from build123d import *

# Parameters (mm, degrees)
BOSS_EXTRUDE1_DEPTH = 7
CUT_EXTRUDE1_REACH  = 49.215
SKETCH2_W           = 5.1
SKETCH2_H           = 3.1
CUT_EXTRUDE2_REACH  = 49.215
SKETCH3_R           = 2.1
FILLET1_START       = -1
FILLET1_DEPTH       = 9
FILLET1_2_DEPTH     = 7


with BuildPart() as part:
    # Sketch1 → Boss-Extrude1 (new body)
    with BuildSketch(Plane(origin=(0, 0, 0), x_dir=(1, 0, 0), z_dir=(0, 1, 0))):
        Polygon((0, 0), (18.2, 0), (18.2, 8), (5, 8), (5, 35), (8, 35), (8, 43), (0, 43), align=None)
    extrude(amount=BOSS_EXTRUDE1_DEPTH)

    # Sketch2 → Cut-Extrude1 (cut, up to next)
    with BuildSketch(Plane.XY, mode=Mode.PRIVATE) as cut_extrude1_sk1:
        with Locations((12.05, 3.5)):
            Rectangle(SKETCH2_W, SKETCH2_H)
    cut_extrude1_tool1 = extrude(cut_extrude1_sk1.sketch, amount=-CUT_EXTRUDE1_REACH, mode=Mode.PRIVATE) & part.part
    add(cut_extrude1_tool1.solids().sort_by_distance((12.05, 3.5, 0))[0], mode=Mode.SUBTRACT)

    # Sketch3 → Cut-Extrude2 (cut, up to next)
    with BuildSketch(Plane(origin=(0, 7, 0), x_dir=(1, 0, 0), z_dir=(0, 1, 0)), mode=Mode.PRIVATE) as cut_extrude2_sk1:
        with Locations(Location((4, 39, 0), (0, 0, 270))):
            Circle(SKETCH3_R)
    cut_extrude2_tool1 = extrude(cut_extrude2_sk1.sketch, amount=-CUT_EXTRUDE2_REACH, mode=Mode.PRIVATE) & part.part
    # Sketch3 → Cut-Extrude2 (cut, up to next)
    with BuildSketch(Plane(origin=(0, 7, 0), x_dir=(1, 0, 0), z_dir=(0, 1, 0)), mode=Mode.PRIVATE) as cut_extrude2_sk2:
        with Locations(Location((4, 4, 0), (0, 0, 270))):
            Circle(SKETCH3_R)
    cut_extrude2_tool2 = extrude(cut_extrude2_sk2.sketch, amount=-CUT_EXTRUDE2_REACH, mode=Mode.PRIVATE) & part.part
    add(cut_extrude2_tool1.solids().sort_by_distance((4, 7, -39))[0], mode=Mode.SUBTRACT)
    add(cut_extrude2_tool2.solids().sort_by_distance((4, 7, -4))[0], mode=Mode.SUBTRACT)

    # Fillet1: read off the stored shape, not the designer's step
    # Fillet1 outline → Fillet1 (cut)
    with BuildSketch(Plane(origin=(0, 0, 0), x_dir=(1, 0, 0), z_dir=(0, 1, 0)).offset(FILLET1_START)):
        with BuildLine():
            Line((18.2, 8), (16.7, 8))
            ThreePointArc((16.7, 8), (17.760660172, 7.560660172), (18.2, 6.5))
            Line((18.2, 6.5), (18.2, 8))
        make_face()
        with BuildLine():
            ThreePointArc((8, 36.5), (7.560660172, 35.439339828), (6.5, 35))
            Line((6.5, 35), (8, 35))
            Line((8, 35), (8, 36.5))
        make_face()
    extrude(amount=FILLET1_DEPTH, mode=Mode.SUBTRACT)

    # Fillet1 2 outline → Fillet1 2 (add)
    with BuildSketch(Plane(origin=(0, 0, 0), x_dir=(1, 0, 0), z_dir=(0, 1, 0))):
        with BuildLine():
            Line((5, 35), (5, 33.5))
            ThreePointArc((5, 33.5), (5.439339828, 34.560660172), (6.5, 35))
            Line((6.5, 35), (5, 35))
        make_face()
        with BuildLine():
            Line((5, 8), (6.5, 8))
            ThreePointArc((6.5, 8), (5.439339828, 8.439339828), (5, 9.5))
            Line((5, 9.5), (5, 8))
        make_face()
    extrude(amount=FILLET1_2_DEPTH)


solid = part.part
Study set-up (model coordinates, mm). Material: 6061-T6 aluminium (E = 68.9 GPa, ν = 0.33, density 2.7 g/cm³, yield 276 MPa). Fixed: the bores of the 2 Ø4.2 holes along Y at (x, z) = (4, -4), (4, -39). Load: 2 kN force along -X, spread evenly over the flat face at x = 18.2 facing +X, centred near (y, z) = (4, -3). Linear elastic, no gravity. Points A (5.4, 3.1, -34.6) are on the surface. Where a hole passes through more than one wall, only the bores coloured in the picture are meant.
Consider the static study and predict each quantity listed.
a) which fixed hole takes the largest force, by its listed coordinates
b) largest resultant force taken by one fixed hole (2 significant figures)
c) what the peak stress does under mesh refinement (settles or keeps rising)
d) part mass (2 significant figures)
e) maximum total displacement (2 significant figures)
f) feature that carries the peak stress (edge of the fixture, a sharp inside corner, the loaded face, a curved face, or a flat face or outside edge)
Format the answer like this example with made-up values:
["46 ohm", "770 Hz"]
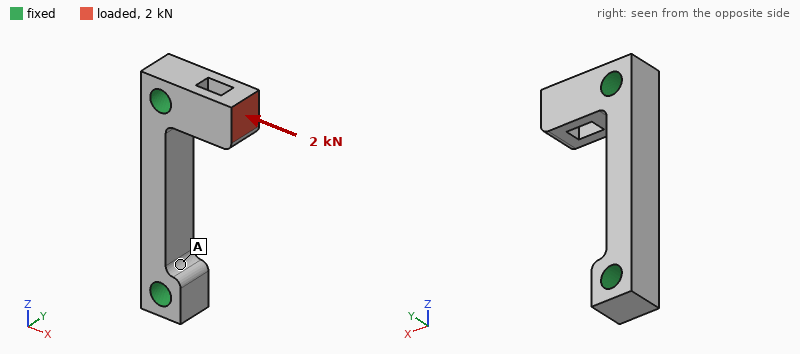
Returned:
["(4, -4)", "2.0 kN", "keeps rising", "5.6 g", "21 µm", "a sharp inside corner"]
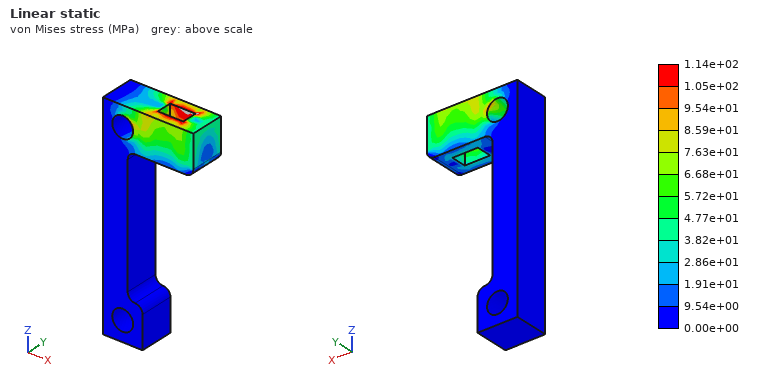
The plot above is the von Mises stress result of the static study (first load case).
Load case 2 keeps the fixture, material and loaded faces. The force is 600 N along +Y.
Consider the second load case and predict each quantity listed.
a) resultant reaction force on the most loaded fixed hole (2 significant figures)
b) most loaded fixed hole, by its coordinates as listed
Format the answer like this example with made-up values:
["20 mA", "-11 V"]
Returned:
["610 N", "(4, -4)"]
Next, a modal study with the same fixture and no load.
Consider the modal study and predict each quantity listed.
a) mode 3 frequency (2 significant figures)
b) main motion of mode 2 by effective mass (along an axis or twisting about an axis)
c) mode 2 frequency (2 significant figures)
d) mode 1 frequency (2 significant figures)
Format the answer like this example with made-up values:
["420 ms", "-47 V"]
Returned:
["27 kHz", "along X", "23 kHz", "22 kHz"]
